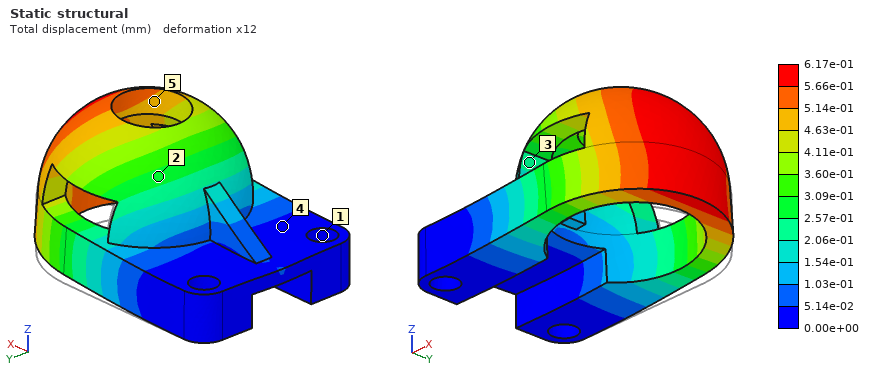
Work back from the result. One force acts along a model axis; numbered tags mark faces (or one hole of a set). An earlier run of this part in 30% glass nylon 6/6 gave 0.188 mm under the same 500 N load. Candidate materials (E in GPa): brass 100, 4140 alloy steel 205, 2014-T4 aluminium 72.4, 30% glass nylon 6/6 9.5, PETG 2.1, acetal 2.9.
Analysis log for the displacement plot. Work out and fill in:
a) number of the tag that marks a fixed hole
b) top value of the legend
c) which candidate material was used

1
6.17e-01 mm
acetal
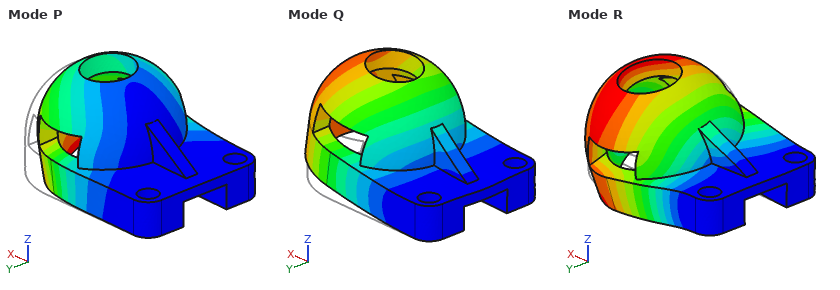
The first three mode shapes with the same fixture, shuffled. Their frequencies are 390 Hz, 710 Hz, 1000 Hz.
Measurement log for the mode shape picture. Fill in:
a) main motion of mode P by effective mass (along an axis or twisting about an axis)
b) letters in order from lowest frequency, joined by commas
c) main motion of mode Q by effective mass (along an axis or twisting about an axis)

along Y
Q, P, R
along Z
